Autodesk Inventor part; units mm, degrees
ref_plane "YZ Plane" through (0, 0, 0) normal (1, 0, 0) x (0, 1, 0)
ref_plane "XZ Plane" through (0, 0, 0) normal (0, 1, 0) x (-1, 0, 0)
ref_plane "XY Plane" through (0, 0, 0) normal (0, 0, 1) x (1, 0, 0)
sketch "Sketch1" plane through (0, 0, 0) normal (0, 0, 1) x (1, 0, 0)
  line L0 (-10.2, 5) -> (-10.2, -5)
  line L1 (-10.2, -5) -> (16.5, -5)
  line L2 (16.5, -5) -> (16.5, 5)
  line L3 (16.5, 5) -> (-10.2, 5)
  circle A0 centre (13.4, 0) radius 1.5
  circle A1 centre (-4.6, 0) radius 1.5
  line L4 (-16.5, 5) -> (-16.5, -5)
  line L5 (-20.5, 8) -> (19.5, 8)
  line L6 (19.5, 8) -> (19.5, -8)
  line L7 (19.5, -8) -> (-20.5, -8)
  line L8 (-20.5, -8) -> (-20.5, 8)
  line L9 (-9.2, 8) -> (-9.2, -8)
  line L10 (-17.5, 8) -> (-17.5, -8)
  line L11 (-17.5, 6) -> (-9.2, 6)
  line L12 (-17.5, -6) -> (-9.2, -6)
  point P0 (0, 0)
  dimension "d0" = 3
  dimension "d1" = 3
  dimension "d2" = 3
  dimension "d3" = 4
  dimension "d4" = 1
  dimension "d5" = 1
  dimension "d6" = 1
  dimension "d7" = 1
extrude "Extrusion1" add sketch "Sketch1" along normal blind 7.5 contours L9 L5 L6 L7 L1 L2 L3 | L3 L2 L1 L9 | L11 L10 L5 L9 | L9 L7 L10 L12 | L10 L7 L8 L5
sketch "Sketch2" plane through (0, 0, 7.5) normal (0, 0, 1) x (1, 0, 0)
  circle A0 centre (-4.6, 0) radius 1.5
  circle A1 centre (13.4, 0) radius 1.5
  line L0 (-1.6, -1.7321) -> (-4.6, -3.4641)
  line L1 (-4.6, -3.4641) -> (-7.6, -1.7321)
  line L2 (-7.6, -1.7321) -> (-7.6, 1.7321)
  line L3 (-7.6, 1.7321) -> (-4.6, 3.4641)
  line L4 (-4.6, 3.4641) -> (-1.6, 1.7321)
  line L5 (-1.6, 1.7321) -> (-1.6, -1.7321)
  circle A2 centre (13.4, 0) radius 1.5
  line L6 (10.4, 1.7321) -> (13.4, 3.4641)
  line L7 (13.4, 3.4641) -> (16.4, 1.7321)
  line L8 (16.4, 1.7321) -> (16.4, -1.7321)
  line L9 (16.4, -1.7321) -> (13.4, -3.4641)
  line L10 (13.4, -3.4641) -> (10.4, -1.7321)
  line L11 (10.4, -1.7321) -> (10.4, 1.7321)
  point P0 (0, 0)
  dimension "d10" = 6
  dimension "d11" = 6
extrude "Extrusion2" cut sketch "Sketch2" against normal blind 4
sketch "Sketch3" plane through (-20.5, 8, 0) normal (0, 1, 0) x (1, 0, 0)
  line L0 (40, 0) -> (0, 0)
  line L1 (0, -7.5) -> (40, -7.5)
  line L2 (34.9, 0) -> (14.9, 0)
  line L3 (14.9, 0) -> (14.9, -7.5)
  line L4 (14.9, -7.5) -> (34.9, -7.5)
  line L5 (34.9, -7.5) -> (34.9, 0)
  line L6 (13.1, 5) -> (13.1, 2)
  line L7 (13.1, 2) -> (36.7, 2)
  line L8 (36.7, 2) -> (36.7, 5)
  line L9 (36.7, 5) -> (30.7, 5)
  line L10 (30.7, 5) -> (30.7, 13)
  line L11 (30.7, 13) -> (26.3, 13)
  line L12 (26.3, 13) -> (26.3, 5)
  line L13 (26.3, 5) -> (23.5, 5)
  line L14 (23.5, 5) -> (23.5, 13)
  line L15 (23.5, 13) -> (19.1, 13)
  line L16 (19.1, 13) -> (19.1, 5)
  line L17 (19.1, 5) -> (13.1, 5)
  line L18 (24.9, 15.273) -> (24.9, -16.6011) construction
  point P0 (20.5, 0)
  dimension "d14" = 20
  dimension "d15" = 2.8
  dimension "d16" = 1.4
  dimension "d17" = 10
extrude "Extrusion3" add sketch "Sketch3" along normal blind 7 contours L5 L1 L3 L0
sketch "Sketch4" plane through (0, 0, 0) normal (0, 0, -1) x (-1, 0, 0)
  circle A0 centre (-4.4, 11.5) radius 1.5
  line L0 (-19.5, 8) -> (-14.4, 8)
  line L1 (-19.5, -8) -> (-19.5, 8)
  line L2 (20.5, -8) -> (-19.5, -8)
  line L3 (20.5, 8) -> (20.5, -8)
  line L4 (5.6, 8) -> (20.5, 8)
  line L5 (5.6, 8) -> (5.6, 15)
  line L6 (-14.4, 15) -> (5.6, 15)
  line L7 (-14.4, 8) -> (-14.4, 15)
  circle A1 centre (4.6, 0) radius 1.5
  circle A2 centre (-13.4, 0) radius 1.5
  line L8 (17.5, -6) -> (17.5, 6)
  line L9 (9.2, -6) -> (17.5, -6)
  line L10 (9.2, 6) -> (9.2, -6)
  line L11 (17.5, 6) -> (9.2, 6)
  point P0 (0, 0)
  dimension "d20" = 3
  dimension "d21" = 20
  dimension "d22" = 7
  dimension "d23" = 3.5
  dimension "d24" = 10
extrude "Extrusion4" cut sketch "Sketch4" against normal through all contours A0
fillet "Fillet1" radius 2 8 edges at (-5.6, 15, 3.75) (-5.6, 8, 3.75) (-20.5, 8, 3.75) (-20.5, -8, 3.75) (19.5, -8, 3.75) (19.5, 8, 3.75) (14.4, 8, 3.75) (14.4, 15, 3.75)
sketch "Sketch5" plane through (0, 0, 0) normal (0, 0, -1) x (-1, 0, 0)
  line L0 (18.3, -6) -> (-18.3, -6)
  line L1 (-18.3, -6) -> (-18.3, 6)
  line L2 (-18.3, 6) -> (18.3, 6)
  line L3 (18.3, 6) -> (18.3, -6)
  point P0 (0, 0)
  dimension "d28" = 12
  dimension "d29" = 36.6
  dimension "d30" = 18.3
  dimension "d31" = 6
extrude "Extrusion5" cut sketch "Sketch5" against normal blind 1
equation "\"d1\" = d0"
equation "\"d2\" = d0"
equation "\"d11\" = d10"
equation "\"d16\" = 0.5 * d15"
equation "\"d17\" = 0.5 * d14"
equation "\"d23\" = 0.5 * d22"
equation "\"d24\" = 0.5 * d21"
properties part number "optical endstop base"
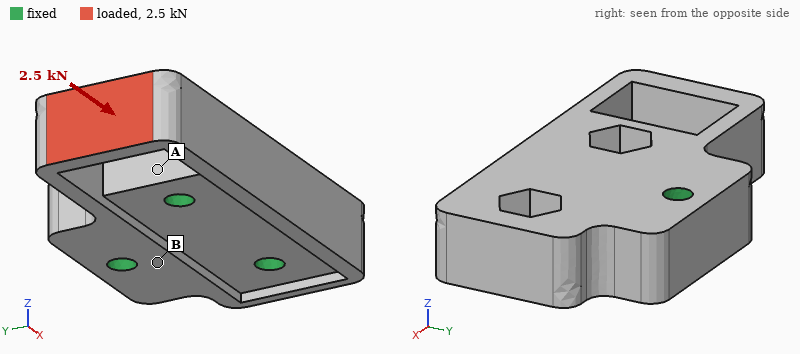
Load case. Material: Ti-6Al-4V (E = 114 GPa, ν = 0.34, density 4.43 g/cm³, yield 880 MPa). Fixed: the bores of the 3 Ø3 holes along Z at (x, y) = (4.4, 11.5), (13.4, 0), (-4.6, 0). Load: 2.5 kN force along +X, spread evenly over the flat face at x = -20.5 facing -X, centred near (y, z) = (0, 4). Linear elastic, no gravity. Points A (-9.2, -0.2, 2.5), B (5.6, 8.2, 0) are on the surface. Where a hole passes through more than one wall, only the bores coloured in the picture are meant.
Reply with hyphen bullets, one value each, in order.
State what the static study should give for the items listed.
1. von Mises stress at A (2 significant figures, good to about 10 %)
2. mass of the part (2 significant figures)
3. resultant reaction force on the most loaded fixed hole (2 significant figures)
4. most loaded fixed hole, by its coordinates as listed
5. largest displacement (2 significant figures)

- 66 MPa
- 19 g
- 1.1 kN
- (-4.6, 0)
- 55 µm
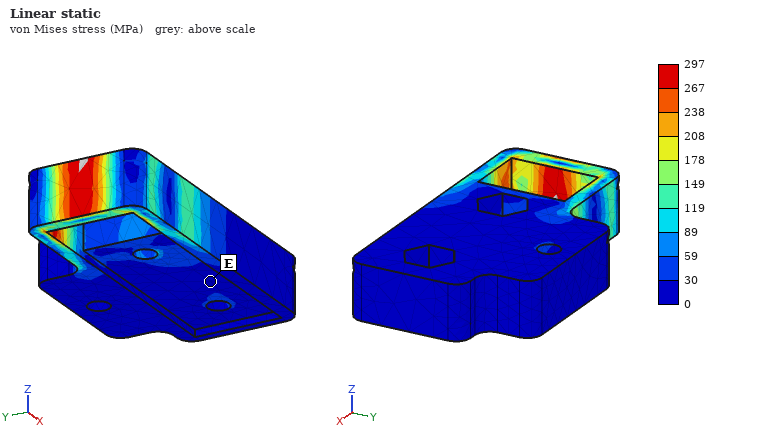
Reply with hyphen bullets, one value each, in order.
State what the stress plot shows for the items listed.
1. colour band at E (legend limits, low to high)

- 0 to 30 MPa
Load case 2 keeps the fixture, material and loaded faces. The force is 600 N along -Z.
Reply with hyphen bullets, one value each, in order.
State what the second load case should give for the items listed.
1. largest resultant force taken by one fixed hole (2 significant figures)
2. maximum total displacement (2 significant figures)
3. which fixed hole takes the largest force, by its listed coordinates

- 1000 N
- 73 µm
- (-4.6, 0)
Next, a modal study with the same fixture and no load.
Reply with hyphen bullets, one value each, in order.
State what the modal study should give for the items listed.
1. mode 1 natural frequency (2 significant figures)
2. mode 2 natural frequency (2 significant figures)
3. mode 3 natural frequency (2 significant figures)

- 11 kHz
- 12 kHz
- 19 kHz
